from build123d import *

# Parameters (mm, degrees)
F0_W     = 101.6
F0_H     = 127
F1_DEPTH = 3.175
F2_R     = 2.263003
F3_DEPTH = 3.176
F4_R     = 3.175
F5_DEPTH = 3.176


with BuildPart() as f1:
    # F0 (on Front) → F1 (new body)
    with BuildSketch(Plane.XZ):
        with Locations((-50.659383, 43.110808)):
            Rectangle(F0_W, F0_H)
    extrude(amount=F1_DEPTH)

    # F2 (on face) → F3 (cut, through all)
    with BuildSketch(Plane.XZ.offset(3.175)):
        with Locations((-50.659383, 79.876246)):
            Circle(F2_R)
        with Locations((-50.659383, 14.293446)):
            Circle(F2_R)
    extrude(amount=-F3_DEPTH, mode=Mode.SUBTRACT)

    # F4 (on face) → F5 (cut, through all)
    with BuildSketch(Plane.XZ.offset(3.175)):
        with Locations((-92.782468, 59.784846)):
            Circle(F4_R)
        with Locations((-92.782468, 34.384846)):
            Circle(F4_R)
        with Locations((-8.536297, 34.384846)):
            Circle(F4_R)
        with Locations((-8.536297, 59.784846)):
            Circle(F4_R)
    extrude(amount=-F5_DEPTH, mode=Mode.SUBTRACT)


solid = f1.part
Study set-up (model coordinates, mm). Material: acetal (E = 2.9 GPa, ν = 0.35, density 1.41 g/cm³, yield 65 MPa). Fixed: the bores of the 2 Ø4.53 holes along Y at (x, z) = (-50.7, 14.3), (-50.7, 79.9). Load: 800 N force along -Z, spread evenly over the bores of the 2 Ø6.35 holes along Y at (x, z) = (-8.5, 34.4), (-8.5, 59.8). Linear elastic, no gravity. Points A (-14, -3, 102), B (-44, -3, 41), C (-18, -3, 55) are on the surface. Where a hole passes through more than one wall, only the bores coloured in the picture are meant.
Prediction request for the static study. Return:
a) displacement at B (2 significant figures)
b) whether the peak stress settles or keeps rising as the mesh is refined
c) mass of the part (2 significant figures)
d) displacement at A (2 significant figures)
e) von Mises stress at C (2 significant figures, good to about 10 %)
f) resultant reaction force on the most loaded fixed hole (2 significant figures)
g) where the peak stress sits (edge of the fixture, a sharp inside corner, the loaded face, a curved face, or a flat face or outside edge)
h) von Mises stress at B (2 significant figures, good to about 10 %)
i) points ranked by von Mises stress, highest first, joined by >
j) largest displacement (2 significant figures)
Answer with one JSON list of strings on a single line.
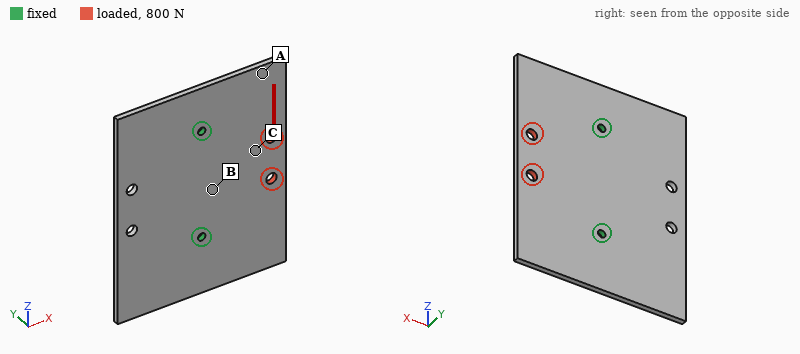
["0.041 mm", "keeps rising", "57 g", "0.17 mm", "6.5 MPa", "650 N", "edge of the fixture", "3.8 MPa", "C > B > A", "0.21 mm"]
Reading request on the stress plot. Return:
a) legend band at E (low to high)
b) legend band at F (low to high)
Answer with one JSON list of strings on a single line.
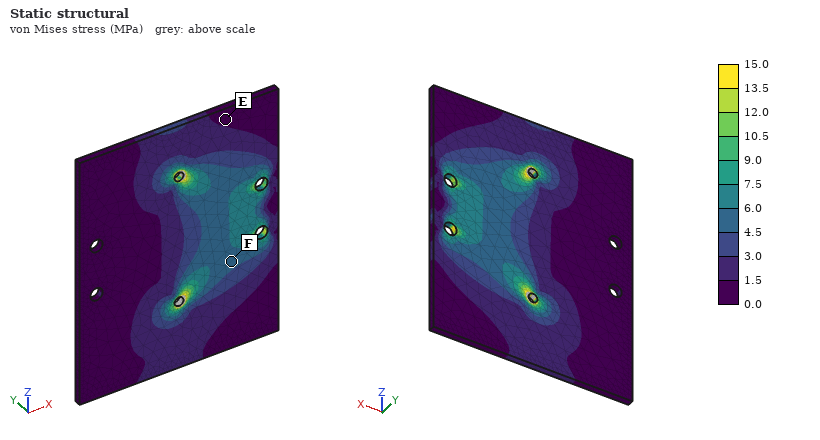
["0.0 to 1.5 MPa", "4.5 to 6.0 MPa"]
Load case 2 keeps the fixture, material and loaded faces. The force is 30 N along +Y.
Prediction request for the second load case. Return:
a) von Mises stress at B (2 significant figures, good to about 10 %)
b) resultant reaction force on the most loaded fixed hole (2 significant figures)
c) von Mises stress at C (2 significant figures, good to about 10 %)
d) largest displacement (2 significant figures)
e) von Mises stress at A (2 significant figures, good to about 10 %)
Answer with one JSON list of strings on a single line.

["3.8 MPa", "15 N", "2.9 MPa", "1.7 mm", "1.6 MPa"]
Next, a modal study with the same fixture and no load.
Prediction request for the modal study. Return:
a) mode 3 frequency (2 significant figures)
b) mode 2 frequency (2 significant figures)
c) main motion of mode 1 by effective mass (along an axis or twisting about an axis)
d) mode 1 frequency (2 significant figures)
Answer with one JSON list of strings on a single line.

["300 Hz", "300 Hz", "twisting about Z", "210 Hz"]
